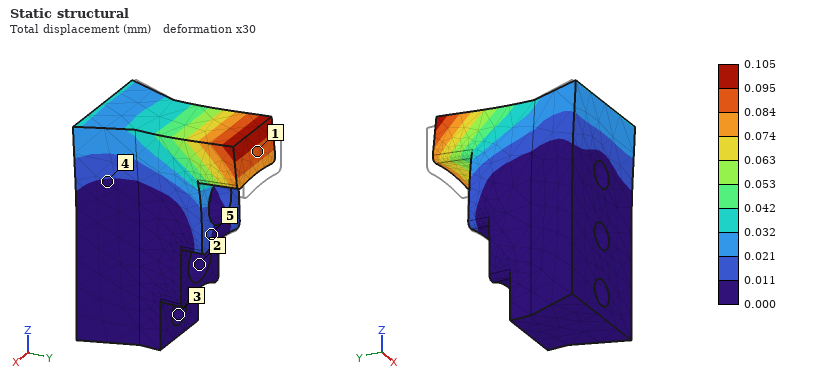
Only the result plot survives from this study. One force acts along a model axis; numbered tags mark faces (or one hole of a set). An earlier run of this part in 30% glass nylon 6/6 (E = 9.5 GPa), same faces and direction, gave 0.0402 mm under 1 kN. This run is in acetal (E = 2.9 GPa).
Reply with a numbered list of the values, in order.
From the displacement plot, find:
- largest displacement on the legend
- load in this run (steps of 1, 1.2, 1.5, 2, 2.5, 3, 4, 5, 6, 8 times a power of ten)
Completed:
1. 0.105 mm
2. 800 N
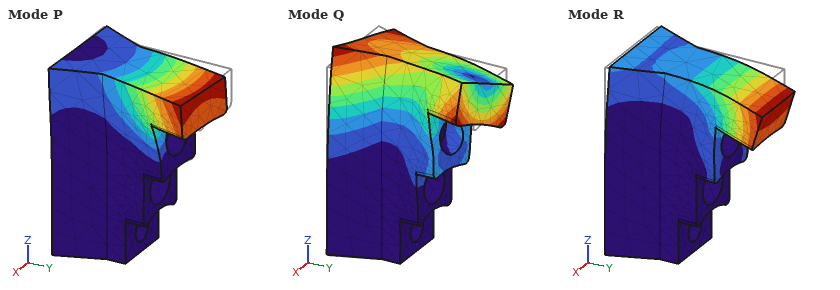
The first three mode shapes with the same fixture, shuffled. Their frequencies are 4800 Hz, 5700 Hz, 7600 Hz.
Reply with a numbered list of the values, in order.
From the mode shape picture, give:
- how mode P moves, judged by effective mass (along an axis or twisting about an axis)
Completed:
1. along X
